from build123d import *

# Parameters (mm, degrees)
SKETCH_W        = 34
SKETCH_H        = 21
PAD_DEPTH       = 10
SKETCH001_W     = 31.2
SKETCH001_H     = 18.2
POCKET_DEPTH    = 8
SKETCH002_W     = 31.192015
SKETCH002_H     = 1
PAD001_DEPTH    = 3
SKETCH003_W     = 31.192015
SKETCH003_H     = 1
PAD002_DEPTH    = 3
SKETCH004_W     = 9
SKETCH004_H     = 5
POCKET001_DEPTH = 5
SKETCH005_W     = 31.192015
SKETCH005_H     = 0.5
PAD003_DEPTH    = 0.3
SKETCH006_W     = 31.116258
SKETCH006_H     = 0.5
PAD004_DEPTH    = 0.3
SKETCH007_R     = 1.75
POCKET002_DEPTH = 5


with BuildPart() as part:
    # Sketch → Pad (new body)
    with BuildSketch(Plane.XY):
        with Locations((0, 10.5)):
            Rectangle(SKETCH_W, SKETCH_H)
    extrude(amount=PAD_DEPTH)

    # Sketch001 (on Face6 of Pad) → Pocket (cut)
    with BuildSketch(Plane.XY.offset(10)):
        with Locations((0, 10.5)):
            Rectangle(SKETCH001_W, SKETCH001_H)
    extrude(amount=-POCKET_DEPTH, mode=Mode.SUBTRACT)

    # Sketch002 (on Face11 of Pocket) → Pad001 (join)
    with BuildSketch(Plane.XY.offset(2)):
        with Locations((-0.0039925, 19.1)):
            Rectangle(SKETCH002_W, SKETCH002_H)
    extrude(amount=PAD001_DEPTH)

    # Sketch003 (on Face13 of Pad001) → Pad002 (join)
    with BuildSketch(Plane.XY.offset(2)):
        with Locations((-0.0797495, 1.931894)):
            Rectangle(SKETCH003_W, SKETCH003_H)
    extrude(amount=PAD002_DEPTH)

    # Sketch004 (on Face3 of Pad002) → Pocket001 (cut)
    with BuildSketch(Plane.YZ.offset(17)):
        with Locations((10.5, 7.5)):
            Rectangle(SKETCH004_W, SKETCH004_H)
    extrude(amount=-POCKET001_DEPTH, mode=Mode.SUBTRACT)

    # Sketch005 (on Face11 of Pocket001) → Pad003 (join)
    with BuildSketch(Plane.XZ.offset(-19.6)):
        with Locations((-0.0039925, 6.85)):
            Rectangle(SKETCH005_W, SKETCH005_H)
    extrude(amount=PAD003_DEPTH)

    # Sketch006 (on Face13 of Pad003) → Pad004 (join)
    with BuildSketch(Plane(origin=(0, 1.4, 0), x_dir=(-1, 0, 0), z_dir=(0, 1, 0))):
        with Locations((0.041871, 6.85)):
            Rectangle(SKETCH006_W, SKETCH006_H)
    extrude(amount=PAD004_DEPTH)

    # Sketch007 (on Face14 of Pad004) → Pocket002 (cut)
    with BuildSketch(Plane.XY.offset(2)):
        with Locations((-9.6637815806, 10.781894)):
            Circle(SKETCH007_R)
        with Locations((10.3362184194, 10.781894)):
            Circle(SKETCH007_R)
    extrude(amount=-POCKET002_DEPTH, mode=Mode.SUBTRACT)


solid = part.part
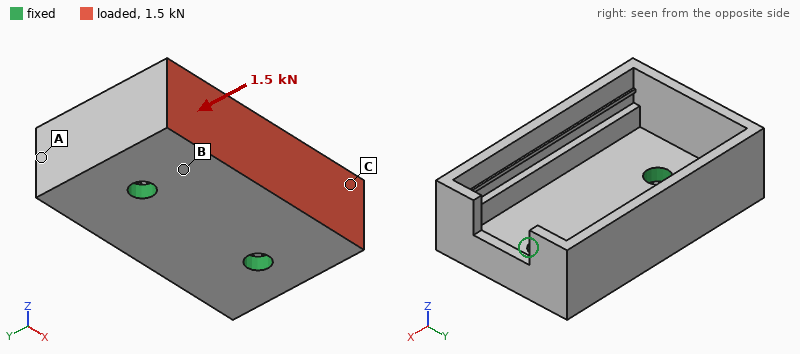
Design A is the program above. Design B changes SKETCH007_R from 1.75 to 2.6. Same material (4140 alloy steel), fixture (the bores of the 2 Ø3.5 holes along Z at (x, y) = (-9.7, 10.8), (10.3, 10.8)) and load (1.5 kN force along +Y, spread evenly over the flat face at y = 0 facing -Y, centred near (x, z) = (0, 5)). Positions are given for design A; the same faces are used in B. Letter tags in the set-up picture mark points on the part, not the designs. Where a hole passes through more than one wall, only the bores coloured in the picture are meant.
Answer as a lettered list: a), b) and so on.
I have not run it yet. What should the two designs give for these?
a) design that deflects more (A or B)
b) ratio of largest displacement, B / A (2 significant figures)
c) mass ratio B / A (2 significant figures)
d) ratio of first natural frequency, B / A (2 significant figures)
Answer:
a) A
b) 0.90
c) 0.98
d) 1.3
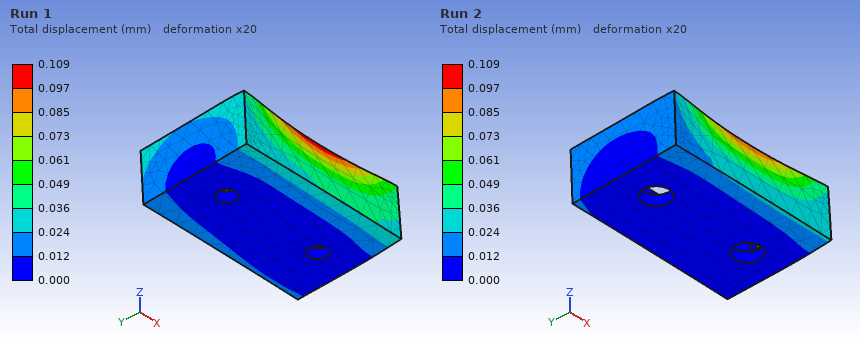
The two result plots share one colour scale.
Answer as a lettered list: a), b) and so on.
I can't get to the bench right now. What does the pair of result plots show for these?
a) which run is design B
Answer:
a) Run 2
